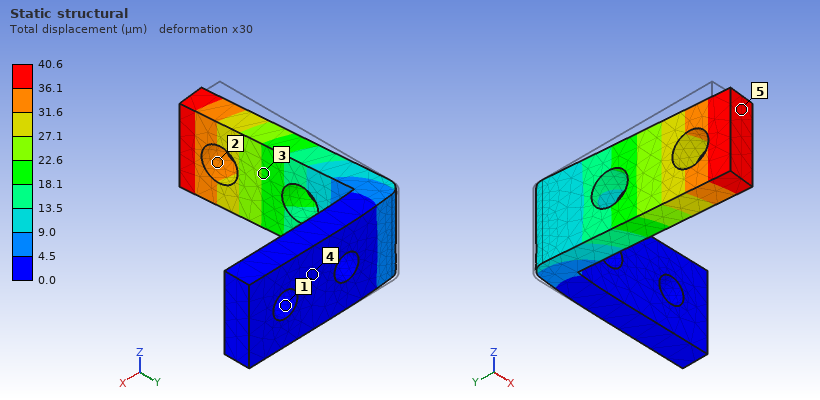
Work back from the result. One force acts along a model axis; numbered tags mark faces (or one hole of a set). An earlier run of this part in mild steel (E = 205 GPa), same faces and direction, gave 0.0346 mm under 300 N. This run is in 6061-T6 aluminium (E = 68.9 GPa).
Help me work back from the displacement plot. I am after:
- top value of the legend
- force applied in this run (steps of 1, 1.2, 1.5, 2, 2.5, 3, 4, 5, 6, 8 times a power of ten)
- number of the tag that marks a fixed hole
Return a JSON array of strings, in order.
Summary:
["40.6 µm", "120 N", "1"]
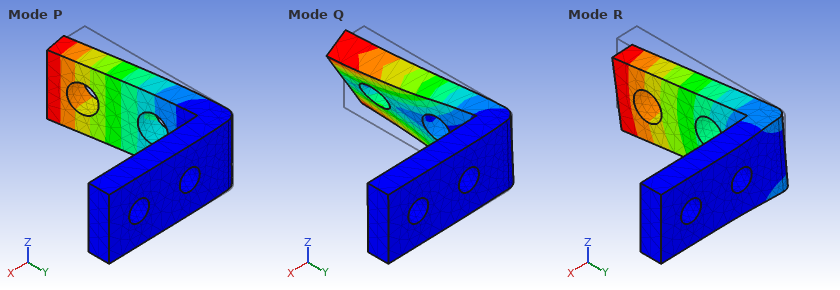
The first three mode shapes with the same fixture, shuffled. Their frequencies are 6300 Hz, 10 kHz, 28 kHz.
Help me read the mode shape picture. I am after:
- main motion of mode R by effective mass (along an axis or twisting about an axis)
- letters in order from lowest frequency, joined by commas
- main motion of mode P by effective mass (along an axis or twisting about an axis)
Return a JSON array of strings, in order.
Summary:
["along Z", "P, R, Q", "along X"]
